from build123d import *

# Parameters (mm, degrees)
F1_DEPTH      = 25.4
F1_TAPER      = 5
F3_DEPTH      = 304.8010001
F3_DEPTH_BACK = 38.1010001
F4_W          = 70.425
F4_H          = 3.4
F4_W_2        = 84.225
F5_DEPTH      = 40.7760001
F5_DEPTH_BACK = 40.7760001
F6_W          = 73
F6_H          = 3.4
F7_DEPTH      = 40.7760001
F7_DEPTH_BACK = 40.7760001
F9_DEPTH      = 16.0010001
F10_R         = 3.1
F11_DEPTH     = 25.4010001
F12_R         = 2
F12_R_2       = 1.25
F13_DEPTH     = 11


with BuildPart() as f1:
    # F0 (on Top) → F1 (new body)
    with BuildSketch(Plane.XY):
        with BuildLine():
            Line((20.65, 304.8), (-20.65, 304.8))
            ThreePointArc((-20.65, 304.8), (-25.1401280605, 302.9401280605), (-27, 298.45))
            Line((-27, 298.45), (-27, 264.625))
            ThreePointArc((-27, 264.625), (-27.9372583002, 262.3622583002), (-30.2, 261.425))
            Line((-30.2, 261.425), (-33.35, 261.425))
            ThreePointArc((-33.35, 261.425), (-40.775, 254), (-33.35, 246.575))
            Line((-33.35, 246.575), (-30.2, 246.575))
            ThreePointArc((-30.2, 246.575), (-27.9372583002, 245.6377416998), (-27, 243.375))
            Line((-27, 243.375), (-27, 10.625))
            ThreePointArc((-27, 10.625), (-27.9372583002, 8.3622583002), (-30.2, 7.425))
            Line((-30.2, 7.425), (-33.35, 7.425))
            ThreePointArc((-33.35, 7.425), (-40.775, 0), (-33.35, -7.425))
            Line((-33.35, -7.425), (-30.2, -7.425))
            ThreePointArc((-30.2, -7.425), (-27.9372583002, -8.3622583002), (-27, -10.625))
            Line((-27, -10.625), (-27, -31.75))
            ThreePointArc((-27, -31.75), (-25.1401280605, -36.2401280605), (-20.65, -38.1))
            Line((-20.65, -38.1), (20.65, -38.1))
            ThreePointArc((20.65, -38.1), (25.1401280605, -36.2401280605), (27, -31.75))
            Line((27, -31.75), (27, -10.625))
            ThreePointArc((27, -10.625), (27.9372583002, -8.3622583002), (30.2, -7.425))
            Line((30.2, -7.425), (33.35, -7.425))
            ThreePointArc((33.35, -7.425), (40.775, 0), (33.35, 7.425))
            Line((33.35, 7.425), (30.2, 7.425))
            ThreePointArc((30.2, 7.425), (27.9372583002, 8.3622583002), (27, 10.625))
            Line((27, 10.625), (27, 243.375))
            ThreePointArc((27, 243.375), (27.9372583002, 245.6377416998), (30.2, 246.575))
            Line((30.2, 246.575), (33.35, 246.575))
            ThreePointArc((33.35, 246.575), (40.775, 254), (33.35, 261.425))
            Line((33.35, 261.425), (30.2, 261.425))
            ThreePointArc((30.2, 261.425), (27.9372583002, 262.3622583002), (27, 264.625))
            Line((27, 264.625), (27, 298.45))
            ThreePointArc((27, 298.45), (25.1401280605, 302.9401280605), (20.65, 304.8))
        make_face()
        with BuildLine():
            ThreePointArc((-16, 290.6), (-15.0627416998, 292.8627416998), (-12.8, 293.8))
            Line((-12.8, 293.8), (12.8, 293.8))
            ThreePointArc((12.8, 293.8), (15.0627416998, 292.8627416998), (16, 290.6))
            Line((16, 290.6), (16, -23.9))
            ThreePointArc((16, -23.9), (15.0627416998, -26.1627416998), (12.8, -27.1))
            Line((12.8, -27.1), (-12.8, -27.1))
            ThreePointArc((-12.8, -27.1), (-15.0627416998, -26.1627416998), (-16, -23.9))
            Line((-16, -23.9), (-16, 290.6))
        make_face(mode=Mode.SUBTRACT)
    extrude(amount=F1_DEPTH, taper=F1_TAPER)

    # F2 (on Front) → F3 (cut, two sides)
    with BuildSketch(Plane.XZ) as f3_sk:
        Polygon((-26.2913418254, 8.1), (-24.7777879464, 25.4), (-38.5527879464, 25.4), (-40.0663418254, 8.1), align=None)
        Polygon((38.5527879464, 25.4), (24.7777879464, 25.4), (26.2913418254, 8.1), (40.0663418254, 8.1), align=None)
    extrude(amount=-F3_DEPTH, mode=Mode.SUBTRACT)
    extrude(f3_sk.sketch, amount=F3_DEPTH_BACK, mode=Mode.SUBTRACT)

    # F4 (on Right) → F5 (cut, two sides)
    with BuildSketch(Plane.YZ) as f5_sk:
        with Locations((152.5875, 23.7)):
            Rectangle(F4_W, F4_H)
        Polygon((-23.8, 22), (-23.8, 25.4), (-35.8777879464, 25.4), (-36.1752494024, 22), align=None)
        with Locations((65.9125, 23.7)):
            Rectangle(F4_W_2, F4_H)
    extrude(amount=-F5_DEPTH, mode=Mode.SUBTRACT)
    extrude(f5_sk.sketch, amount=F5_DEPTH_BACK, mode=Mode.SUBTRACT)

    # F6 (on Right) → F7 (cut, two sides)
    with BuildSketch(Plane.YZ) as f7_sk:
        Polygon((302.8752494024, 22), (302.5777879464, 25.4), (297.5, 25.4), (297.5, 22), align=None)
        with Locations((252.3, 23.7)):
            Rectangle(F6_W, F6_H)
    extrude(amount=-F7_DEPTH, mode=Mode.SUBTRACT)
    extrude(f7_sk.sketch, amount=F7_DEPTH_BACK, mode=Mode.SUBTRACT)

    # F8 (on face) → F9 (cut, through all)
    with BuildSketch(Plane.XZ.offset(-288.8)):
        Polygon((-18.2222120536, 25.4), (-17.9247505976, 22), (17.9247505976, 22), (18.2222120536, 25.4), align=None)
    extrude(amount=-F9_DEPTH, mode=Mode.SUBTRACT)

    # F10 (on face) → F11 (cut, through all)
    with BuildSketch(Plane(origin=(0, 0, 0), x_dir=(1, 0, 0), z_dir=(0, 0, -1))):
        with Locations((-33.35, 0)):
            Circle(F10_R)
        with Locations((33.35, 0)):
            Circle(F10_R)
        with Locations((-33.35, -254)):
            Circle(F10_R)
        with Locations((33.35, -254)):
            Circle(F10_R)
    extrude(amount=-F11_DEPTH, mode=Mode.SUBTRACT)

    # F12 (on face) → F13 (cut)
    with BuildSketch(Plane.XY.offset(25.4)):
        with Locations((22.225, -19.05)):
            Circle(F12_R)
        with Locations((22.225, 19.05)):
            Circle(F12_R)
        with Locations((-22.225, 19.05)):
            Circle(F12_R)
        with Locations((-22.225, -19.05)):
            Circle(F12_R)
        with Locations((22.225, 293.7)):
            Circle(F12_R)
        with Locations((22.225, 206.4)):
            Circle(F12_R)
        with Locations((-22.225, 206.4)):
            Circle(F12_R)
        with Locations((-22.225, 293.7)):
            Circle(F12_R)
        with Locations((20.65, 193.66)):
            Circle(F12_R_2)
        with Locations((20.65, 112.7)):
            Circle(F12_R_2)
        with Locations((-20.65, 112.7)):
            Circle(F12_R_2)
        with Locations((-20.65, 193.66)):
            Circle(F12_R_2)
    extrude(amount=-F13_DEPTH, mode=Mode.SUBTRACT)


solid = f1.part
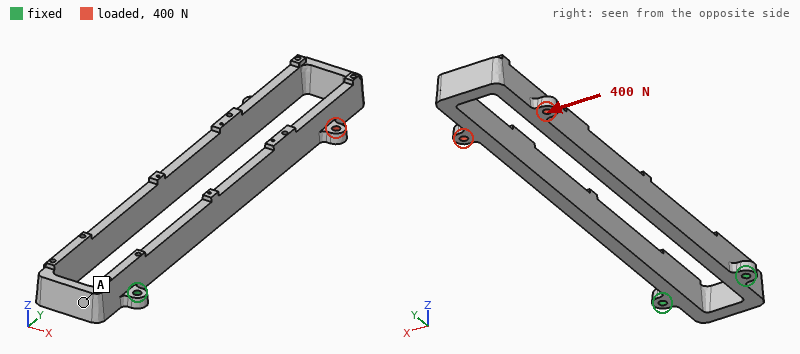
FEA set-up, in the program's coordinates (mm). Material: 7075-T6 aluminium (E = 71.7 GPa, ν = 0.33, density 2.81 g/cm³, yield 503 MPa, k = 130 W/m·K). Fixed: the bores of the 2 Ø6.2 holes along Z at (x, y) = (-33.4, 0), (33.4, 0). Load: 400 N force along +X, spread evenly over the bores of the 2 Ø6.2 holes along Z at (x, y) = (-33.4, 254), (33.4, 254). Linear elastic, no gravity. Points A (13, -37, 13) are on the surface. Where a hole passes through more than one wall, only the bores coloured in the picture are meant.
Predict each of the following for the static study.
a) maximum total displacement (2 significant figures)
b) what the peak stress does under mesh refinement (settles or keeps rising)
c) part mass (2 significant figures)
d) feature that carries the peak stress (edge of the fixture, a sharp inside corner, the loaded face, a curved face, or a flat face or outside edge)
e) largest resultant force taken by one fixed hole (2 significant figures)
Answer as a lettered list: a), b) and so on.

a) 4.2 mm
b) keeps rising
c) 440 g
d) a sharp inside corner
e) 1.2 kN
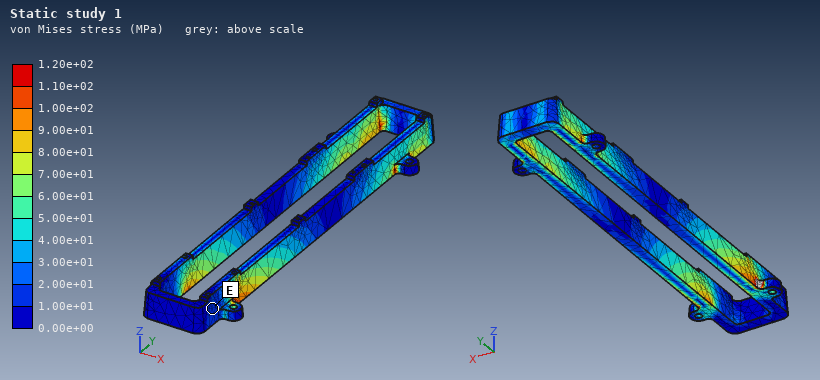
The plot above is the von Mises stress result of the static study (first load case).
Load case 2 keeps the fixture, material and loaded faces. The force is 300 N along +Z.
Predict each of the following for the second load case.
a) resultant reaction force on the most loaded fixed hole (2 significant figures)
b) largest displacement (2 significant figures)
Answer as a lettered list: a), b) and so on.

a) 170 N
b) 3.4 mm
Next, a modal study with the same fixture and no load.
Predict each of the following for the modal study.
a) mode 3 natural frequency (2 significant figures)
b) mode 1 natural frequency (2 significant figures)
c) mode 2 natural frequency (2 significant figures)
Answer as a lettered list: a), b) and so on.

a) 490 Hz
b) 120 Hz
c) 120 Hz
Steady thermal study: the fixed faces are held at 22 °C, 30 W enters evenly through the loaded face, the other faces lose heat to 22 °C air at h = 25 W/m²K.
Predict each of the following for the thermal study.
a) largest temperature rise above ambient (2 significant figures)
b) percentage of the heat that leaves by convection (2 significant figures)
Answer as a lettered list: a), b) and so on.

a) 58 K
b) 85 %
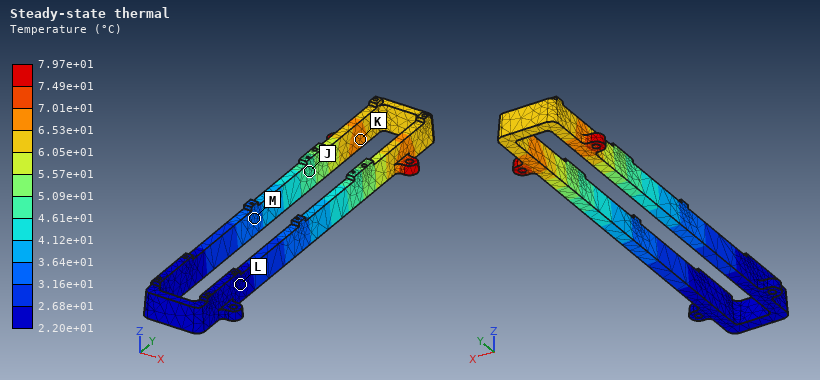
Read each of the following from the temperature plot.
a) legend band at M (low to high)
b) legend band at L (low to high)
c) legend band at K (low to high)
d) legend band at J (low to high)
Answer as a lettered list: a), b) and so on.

a) 3.16e+01 to 3.64e+01 °C
b) 2.20e+01 to 2.68e+01 °C
c) 6.53e+01 to 7.01e+01 °C
d) 4.61e+01 to 5.09e+01 °C
